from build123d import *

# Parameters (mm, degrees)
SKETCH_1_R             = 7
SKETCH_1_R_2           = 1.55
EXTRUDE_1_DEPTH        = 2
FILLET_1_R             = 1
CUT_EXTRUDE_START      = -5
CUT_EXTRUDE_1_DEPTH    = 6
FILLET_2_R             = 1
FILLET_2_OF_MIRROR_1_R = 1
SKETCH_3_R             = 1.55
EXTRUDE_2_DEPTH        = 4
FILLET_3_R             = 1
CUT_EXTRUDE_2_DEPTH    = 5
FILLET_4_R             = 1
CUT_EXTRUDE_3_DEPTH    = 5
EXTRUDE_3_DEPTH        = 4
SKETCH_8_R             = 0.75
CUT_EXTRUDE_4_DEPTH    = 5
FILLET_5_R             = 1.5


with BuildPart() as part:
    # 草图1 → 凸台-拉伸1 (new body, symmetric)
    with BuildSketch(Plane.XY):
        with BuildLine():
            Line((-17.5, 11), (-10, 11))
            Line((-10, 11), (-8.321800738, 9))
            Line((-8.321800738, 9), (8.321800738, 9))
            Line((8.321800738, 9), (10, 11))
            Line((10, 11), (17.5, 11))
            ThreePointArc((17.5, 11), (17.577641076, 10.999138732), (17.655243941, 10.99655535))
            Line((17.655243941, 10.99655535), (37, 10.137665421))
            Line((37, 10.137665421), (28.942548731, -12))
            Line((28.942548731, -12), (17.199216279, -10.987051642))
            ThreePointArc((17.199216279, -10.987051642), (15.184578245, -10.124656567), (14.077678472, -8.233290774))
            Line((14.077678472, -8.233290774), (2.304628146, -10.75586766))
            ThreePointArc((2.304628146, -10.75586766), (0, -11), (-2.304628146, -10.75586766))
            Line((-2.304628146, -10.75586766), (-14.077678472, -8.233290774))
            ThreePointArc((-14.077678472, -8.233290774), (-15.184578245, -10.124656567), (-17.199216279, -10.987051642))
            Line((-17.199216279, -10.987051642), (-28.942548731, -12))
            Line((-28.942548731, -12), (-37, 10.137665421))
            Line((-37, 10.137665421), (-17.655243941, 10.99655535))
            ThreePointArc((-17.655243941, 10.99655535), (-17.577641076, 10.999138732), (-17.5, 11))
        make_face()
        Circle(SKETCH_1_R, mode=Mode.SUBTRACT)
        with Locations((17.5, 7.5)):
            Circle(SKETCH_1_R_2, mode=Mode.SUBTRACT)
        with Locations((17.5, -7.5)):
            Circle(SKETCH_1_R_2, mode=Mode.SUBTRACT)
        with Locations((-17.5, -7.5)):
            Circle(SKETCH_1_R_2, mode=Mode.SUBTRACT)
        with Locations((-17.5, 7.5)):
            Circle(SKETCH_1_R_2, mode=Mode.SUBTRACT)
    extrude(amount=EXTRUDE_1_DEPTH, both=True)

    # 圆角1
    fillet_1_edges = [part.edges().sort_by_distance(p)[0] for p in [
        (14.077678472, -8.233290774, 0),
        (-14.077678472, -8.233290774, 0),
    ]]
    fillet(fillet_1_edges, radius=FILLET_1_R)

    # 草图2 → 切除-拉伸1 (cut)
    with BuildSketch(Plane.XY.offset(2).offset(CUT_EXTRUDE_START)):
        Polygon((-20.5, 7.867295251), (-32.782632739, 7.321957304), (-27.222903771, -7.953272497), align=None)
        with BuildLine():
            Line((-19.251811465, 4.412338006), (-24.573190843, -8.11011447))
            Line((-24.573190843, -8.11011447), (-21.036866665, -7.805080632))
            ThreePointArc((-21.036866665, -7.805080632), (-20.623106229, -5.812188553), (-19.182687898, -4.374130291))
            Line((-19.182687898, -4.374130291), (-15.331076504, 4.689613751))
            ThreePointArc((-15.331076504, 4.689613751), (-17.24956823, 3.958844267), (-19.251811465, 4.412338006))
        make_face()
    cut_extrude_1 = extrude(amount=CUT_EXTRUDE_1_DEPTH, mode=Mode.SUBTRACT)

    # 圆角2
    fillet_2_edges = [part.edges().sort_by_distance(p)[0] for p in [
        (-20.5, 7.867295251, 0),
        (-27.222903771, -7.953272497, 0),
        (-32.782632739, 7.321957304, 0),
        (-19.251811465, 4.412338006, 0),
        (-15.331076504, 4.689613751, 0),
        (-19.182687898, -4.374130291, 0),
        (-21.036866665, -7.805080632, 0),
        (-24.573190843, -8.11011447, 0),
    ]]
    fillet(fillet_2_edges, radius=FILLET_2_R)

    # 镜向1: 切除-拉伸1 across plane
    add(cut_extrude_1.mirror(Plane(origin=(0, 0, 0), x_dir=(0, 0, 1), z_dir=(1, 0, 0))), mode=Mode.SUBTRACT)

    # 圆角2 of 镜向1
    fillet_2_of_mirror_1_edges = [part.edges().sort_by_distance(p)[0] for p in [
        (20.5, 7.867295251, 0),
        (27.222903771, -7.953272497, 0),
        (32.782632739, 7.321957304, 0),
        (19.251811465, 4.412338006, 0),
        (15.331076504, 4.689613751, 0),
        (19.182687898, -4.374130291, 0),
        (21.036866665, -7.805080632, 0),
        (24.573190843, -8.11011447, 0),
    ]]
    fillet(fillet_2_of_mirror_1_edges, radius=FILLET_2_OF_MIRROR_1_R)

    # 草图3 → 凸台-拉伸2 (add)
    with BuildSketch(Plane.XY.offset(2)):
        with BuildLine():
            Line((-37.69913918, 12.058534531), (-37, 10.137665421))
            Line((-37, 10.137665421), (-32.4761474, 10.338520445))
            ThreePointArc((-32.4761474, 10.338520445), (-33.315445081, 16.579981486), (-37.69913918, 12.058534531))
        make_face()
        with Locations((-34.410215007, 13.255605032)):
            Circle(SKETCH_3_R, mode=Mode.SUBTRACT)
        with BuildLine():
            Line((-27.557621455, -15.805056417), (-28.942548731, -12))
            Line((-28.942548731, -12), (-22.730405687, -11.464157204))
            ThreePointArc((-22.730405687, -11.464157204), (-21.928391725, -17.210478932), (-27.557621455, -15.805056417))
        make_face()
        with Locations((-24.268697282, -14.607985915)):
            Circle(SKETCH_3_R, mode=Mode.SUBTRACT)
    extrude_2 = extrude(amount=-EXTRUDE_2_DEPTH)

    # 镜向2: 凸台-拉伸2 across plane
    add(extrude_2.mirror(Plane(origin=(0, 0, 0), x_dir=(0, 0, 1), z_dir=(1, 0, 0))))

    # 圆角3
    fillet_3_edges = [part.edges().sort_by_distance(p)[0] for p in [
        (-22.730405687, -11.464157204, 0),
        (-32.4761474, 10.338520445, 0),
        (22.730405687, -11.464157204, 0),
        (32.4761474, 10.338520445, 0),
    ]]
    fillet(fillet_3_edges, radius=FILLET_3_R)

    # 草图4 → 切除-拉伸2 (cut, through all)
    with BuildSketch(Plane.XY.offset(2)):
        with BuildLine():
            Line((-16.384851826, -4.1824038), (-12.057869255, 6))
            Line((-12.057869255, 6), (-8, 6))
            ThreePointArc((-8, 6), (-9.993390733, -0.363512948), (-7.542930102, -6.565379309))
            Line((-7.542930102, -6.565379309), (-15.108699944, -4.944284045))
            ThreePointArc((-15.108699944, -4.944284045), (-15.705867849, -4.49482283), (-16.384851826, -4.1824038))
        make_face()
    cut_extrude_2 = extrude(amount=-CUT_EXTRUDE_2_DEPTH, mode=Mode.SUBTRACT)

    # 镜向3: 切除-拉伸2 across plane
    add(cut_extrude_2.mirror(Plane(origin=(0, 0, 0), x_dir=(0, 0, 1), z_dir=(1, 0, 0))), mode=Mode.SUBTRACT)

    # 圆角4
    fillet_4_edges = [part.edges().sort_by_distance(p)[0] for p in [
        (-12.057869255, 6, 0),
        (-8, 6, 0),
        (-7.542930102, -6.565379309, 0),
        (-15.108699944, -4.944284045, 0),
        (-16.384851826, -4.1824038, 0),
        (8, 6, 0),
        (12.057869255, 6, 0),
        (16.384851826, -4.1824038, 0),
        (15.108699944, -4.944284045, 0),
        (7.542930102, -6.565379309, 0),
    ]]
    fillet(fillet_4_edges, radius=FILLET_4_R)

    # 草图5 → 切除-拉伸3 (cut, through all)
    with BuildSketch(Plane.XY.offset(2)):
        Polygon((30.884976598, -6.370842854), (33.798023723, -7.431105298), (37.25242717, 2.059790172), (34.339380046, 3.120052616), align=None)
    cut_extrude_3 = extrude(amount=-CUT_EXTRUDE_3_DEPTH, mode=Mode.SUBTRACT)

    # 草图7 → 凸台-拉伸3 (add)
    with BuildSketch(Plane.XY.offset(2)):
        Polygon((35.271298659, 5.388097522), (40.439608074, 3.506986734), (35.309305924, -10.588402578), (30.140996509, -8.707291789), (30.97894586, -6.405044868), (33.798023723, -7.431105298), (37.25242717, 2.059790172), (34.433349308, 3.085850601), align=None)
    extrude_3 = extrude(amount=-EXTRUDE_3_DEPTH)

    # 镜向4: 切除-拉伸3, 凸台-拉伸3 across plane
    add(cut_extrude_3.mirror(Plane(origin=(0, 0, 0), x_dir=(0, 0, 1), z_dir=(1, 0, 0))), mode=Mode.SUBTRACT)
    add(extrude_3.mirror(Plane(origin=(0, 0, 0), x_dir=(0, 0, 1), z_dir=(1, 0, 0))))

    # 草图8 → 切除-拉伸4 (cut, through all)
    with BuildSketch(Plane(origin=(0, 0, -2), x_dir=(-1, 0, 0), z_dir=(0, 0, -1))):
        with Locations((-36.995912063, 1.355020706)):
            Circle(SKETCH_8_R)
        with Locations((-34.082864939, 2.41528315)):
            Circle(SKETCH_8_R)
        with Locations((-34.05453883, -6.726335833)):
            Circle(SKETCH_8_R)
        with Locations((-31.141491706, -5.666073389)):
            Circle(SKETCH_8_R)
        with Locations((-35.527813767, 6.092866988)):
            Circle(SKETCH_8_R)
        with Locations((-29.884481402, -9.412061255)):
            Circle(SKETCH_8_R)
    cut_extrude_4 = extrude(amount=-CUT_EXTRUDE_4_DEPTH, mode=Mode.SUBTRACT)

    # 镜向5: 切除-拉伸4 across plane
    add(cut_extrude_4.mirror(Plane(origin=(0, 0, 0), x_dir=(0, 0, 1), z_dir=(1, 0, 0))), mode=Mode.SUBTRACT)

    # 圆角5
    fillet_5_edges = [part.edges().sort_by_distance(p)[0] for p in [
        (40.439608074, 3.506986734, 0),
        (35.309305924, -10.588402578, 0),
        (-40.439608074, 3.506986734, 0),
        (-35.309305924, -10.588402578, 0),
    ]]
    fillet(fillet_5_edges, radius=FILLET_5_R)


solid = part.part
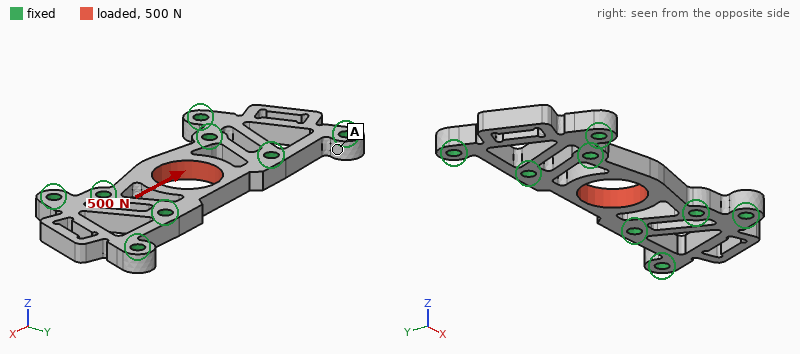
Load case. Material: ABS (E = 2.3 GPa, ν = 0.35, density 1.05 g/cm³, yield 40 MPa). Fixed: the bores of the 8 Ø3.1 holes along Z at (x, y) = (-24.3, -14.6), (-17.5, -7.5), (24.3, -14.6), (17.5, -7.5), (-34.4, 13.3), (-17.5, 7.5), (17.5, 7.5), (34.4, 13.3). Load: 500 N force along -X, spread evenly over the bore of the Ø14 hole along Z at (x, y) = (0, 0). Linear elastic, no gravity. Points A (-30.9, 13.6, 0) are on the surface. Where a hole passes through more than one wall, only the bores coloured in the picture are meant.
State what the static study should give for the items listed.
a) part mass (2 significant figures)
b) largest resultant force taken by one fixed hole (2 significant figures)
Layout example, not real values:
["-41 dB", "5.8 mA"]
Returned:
["4.4 g", "130 N"]
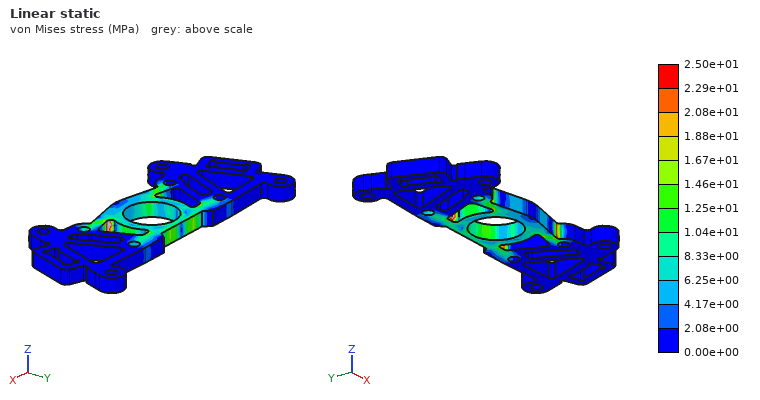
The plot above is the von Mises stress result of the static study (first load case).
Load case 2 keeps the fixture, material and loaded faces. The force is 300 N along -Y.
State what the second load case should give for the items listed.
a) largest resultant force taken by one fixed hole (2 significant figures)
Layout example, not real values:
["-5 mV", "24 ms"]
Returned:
["100 N"]
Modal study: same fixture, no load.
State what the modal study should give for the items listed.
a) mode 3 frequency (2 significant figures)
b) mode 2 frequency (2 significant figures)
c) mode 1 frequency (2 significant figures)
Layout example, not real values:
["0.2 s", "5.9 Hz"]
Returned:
["4600 Hz", "4600 Hz", "4600 Hz"]
